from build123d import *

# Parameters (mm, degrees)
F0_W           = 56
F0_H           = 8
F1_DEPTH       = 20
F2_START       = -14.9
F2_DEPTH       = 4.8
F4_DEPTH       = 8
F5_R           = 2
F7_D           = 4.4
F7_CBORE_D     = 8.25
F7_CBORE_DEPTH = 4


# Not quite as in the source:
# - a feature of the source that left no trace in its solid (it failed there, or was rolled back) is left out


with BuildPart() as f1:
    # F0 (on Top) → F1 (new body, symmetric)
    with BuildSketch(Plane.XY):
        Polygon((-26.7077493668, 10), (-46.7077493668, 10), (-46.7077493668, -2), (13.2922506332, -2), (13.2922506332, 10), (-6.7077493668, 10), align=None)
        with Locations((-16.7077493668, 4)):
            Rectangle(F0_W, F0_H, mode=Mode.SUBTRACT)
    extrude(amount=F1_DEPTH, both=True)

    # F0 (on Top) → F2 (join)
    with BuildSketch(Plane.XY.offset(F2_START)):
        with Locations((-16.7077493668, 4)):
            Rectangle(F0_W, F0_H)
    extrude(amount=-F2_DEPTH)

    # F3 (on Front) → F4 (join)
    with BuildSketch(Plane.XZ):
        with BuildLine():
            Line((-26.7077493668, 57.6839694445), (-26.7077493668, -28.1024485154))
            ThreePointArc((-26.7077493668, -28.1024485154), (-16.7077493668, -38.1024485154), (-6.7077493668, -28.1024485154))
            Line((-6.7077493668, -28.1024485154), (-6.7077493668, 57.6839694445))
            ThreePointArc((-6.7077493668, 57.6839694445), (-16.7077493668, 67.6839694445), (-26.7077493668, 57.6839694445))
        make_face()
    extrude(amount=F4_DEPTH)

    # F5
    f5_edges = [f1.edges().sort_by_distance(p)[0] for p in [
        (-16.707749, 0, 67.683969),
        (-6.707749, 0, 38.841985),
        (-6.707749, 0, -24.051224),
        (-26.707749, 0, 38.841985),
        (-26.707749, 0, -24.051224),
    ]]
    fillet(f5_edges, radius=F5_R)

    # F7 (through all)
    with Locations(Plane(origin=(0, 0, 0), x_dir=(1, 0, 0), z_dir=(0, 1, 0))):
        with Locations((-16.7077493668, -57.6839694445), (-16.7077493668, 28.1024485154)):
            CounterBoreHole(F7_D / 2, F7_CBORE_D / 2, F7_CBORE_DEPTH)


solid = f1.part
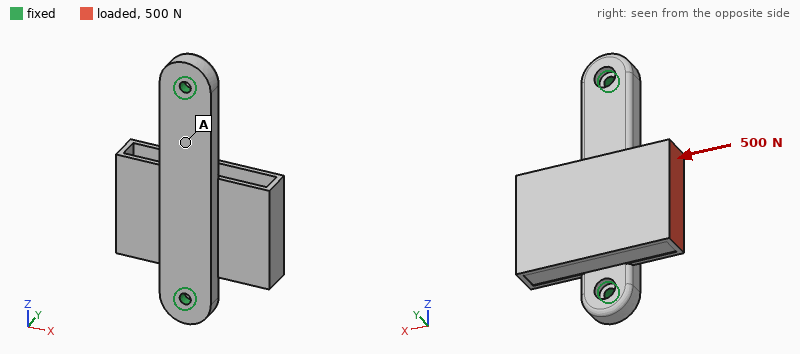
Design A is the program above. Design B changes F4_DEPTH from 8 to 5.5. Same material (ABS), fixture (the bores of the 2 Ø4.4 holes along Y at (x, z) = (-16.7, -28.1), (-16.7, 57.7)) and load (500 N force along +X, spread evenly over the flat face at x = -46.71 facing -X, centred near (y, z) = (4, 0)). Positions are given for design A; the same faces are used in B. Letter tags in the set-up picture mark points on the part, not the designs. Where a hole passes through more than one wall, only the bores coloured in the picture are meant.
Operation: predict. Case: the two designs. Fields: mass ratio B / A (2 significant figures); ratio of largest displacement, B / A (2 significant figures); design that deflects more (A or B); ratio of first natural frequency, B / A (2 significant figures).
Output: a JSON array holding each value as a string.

["0.81", "3.3", "B", "0.57"]
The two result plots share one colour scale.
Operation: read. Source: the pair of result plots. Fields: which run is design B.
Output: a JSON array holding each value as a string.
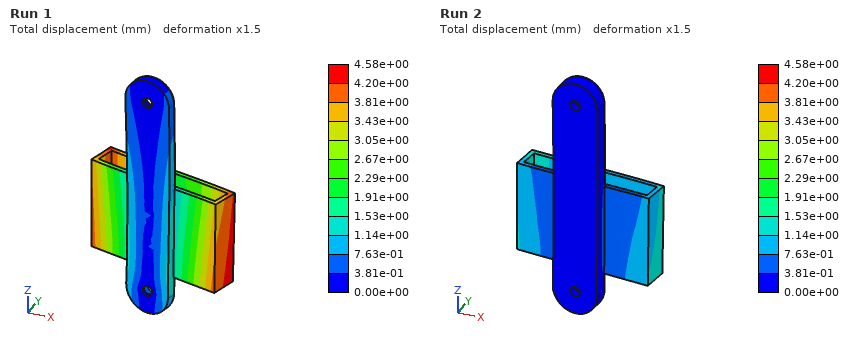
["Run 1"]
